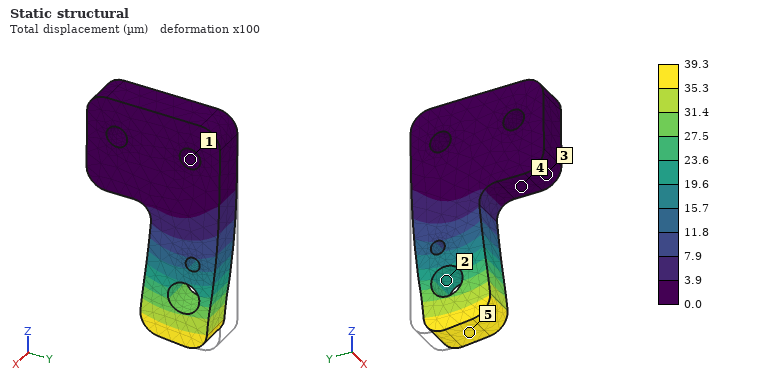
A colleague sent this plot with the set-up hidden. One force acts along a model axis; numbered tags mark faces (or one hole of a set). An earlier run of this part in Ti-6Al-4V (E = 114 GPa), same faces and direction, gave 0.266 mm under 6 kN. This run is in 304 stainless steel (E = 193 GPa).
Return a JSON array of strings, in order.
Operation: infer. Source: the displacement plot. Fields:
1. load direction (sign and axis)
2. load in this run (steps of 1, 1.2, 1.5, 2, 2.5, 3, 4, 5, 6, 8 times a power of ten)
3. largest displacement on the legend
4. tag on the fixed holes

["-Y", "1.5 kN", "39.3 µm", "1"]
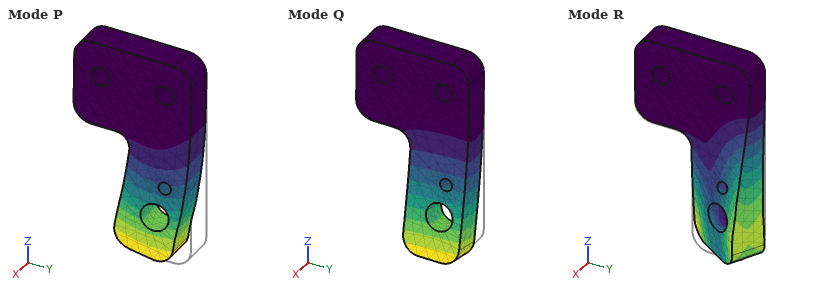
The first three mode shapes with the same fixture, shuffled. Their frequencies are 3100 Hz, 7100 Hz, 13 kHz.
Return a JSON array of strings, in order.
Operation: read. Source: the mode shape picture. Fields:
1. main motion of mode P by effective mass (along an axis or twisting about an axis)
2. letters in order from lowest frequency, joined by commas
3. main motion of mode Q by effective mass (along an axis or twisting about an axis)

["along Y", "Q, P, R", "along X"]
